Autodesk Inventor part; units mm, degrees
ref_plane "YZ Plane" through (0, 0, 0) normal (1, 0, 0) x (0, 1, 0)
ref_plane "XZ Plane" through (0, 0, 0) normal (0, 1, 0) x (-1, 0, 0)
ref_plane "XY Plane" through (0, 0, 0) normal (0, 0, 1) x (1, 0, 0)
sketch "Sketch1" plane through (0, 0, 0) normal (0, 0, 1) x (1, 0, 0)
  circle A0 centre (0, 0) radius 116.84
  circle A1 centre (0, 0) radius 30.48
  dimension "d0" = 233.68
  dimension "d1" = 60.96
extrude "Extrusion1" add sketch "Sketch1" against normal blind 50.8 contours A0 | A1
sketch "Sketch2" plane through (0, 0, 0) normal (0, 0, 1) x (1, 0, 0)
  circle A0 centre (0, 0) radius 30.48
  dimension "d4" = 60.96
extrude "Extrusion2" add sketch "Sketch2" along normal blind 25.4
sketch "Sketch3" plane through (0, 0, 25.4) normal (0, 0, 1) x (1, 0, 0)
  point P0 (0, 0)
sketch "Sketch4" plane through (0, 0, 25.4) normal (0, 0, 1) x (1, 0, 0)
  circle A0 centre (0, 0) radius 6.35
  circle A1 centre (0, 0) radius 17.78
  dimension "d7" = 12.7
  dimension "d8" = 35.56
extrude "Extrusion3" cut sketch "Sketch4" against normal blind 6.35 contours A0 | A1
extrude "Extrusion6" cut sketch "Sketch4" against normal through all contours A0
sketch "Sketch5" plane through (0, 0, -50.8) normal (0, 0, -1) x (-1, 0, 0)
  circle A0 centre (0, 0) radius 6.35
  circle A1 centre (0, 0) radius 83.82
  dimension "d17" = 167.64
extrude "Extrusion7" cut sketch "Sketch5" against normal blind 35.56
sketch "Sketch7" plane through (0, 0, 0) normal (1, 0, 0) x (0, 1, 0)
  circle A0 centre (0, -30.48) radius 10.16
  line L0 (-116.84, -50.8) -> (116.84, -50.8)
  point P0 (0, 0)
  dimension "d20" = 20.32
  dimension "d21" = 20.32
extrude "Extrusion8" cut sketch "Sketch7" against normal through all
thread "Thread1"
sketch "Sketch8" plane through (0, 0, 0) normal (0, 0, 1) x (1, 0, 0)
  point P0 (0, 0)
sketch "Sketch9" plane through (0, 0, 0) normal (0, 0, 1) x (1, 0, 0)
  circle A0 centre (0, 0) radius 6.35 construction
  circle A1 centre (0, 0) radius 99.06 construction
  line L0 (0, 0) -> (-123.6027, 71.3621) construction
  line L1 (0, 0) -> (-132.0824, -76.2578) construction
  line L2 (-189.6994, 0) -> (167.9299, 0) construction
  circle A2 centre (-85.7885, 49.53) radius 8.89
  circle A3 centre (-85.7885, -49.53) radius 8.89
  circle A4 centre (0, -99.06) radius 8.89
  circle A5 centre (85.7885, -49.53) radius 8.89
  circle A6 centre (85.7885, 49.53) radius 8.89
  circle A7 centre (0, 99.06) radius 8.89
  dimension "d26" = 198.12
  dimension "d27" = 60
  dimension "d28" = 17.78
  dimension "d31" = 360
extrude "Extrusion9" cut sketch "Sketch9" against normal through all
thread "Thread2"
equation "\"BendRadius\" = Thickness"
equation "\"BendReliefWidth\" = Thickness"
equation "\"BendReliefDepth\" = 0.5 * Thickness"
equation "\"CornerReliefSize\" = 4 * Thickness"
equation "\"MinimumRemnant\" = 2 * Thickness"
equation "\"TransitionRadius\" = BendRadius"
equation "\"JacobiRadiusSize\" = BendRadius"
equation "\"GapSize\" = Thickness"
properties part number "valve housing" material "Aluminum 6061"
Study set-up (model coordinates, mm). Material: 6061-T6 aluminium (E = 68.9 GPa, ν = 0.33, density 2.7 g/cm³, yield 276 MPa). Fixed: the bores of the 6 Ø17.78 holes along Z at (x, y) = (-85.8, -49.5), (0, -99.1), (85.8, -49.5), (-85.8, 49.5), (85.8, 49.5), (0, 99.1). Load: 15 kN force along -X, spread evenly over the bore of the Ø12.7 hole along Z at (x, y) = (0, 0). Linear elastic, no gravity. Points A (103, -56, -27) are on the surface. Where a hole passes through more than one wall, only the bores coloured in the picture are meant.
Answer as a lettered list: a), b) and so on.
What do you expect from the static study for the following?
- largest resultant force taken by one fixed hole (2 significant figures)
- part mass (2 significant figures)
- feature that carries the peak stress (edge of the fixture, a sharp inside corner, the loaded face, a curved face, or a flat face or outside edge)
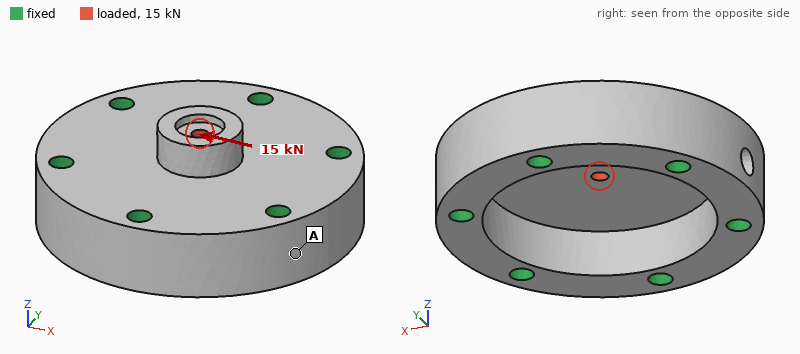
a) 3.5 kN
b) 3.7 kg
c) the loaded face
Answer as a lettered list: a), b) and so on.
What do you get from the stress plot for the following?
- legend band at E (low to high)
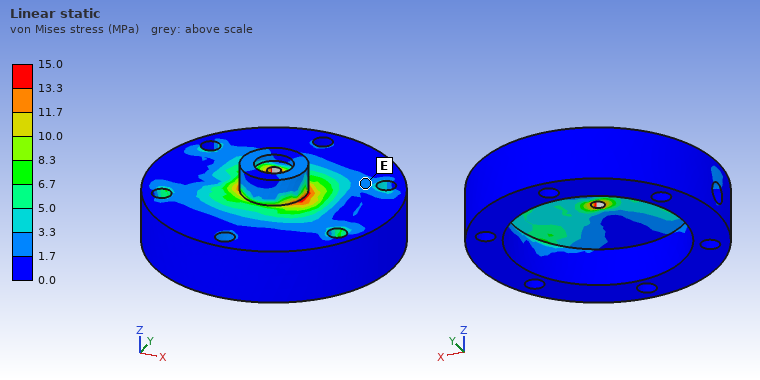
a) 1.7 to 3.3 MPa
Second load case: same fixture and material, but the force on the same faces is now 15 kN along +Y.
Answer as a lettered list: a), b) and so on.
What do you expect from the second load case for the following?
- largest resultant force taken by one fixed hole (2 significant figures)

a) 3.9 kN
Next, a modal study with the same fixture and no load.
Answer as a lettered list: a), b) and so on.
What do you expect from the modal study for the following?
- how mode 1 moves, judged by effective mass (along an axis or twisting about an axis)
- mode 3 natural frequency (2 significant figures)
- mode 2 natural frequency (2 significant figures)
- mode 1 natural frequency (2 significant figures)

a) along Z
b) 6800 Hz
c) 6800 Hz
d) 3800 Hz
